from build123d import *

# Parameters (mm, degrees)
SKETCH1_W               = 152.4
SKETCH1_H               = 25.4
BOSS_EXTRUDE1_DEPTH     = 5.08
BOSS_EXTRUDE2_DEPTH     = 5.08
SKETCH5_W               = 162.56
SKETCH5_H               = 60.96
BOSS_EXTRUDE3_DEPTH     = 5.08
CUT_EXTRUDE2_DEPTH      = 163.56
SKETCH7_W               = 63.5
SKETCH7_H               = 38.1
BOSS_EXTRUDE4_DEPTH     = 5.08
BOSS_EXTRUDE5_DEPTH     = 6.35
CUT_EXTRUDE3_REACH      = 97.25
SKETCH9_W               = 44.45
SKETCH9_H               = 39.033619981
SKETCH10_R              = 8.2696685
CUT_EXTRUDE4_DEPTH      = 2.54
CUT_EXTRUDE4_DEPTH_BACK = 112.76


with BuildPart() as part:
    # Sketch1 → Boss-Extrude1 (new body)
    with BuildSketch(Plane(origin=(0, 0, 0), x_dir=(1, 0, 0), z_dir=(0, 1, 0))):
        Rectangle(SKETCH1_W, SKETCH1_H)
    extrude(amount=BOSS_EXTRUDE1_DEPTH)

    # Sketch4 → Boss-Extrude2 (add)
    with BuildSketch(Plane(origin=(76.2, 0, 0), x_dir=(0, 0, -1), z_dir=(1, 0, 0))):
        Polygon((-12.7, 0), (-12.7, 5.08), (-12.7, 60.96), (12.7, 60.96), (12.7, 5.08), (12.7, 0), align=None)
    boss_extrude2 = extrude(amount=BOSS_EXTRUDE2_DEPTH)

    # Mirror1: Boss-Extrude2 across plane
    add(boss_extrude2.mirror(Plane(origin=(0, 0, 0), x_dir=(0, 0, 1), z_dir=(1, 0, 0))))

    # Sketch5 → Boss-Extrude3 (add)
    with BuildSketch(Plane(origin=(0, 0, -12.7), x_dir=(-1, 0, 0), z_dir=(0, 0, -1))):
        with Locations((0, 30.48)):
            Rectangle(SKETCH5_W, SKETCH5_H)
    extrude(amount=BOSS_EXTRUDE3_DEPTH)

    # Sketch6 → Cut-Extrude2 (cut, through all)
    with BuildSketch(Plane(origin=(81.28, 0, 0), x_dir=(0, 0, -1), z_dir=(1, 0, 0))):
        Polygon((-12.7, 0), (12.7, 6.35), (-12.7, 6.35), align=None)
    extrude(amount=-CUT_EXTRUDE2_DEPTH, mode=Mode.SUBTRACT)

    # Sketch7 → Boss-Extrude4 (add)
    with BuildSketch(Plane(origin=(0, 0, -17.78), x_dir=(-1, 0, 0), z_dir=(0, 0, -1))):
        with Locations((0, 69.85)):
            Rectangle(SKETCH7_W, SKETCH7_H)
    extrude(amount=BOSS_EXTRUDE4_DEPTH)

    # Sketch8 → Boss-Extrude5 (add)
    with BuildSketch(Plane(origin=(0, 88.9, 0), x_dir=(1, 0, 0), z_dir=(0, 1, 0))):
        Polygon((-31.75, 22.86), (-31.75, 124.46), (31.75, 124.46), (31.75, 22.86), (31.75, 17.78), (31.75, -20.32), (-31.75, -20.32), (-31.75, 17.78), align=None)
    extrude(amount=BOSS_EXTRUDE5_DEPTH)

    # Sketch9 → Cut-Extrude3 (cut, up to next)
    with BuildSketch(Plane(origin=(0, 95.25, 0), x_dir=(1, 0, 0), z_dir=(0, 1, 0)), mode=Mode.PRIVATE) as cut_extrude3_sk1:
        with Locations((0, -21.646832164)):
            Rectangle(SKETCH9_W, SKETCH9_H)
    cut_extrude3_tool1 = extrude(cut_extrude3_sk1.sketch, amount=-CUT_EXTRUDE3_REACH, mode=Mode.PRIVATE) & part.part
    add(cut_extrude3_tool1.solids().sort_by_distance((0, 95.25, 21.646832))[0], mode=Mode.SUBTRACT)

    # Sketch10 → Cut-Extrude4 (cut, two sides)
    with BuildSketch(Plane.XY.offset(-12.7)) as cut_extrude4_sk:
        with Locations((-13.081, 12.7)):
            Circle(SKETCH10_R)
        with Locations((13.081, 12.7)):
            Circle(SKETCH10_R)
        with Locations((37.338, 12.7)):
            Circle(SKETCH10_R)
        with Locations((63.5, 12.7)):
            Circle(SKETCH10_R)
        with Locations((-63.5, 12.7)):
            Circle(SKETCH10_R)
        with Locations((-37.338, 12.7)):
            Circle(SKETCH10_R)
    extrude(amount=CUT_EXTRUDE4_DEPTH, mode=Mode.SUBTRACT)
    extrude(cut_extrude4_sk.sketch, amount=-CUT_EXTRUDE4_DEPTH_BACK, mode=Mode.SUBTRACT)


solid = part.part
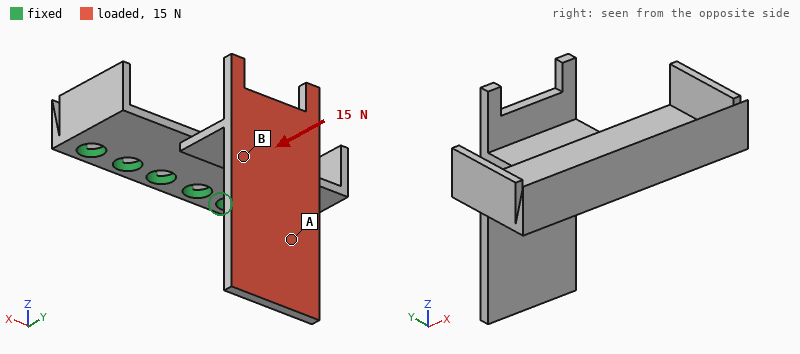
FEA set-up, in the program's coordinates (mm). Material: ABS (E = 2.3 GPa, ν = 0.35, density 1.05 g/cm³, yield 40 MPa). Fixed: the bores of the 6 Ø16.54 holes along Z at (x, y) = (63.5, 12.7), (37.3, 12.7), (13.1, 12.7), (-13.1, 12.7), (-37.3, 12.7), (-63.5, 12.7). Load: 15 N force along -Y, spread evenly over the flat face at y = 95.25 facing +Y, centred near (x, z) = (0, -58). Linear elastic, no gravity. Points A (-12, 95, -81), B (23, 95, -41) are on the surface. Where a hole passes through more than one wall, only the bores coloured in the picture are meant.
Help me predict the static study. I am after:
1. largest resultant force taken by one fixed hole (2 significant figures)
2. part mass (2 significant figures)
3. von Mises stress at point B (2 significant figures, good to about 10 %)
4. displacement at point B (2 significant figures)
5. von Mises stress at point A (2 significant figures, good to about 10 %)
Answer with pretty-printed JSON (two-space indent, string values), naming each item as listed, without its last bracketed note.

{
  "largest resultant force taken by one fixed hole": "8.7 N",
  "part mass": "140 g",
  "von Mises stress at point B": "0.90 MPa",
  "displacement at point B": "0.72 mm",
  "von Mises stress at point A": "0.25 MPa"
}
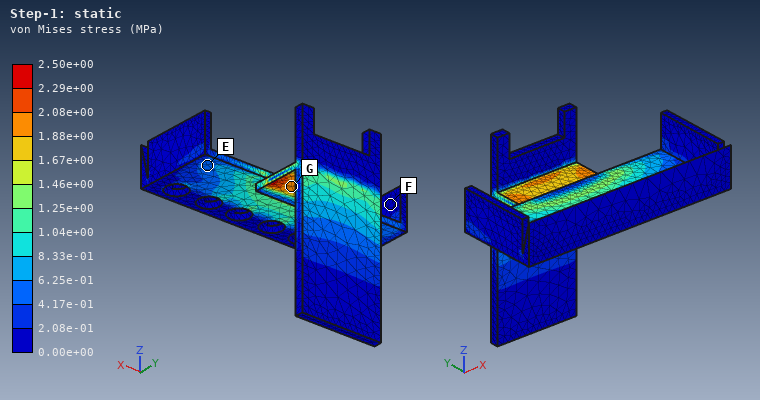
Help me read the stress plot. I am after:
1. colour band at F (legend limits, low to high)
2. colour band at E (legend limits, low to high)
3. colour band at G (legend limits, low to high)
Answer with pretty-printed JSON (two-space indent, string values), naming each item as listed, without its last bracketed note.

{
  "colour band at F": "0.00e+00 to 2.08e-01 MPa",
  "colour band at E": "4.17e-01 to 6.25e-01 MPa",
  "colour band at G": "1.88e+00 to 2.08e+00 MPa"
}
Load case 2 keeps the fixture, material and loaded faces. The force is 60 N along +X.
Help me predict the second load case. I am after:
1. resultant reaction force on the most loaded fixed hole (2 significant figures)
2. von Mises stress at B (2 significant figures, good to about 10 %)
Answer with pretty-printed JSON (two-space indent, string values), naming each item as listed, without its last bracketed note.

{
  "resultant reaction force on the most loaded fixed hole": "32 N",
  "von Mises stress at B": "0.38 MPa"
}
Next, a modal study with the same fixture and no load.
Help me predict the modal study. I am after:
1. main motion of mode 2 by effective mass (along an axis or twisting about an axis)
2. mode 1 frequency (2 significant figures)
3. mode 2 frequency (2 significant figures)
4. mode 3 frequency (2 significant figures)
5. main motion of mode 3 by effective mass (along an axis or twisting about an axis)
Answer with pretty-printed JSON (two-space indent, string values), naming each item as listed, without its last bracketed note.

{
  "main motion of mode 2 by effective mass": "along X",
  "mode 1 frequency": "58 Hz",
  "mode 2 frequency": "120 Hz",
  "mode 3 frequency": "180 Hz",
  "main motion of mode 3 by effective mass": "along Z"
}
